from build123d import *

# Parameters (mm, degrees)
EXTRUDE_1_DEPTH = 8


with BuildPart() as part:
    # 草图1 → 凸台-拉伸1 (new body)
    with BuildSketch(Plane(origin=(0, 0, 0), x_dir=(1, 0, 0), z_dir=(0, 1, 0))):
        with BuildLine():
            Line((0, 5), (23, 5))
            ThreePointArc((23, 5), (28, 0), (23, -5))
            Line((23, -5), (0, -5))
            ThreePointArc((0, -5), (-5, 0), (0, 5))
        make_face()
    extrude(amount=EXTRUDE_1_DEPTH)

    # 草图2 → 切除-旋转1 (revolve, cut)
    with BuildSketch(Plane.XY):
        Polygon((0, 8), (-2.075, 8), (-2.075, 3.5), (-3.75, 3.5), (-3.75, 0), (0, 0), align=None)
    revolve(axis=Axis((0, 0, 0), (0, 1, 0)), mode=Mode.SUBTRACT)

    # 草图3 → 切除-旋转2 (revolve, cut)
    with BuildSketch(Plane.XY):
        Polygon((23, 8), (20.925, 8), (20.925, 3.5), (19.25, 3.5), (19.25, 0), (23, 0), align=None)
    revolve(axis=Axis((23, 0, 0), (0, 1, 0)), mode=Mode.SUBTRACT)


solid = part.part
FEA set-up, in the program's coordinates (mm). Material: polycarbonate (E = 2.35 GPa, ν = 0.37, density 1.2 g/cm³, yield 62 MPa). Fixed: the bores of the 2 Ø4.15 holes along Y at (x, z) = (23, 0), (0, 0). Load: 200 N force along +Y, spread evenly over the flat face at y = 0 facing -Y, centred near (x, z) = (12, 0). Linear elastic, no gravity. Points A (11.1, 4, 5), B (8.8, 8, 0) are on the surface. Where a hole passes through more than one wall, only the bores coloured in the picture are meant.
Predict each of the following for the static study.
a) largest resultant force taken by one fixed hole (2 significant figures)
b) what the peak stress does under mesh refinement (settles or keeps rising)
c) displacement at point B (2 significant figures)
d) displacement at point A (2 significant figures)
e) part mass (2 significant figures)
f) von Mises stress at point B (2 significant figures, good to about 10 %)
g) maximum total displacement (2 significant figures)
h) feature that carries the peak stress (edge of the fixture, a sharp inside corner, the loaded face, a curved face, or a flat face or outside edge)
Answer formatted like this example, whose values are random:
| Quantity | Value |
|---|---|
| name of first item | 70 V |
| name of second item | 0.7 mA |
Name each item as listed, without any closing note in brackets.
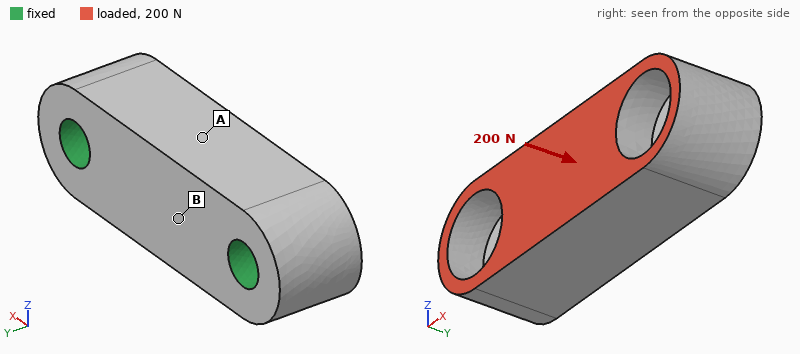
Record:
| Quantity | Value |
|---|---|
| largest resultant force taken by one fixed hole | 110 N |
| what the peak stress does under mesh refinement | keeps rising |
| displacement at point B | 17 µm |
| displacement at point A | 20 µm |
| part mass | 2.4 g |
| von Mises stress at point B | 1.8 MPa |
| maximum total displacement | 20 µm |
| feature that carries the peak stress | edge of the fixture |
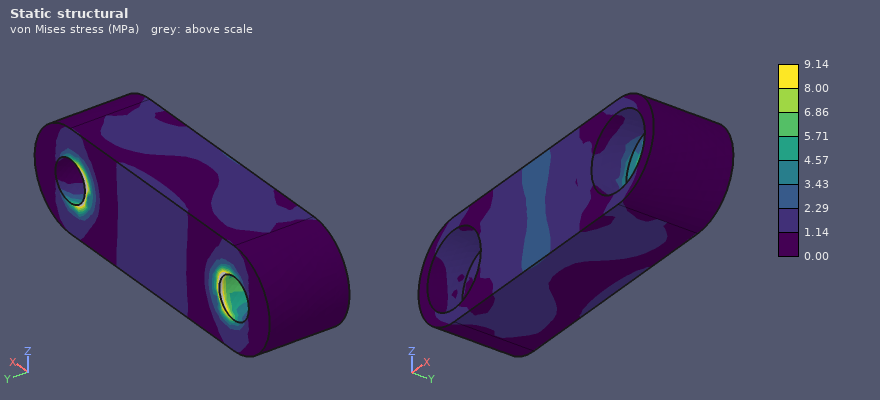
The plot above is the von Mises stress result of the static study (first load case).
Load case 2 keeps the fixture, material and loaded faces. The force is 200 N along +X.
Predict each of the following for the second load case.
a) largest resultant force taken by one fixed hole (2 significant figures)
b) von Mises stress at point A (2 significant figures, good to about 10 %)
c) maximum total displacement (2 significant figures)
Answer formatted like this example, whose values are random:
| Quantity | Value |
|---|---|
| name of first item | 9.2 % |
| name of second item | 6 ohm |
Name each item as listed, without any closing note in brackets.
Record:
| Quantity | Value |
|---|---|
| largest resultant force taken by one fixed hole | 110 N |
| von Mises stress at point A | 1.2 MPa |
| maximum total displacement | 22 µm |
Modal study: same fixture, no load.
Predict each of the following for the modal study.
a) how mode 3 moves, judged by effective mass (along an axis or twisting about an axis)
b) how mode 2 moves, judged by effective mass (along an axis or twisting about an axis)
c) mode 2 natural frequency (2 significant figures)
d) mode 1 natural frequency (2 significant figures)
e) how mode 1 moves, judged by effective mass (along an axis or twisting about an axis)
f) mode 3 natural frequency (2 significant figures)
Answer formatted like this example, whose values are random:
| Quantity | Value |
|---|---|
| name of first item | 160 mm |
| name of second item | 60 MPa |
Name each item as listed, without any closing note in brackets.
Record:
| Quantity | Value |
|---|---|
| how mode 3 moves, judged by effective mass | along Z |
| how mode 2 moves, judged by effective mass | along Y |
| mode 2 natural frequency | 12 kHz |
| mode 1 natural frequency | 10 kHz |
| how mode 1 moves, judged by effective mass | along Z |
| mode 3 natural frequency | 15 kHz |
